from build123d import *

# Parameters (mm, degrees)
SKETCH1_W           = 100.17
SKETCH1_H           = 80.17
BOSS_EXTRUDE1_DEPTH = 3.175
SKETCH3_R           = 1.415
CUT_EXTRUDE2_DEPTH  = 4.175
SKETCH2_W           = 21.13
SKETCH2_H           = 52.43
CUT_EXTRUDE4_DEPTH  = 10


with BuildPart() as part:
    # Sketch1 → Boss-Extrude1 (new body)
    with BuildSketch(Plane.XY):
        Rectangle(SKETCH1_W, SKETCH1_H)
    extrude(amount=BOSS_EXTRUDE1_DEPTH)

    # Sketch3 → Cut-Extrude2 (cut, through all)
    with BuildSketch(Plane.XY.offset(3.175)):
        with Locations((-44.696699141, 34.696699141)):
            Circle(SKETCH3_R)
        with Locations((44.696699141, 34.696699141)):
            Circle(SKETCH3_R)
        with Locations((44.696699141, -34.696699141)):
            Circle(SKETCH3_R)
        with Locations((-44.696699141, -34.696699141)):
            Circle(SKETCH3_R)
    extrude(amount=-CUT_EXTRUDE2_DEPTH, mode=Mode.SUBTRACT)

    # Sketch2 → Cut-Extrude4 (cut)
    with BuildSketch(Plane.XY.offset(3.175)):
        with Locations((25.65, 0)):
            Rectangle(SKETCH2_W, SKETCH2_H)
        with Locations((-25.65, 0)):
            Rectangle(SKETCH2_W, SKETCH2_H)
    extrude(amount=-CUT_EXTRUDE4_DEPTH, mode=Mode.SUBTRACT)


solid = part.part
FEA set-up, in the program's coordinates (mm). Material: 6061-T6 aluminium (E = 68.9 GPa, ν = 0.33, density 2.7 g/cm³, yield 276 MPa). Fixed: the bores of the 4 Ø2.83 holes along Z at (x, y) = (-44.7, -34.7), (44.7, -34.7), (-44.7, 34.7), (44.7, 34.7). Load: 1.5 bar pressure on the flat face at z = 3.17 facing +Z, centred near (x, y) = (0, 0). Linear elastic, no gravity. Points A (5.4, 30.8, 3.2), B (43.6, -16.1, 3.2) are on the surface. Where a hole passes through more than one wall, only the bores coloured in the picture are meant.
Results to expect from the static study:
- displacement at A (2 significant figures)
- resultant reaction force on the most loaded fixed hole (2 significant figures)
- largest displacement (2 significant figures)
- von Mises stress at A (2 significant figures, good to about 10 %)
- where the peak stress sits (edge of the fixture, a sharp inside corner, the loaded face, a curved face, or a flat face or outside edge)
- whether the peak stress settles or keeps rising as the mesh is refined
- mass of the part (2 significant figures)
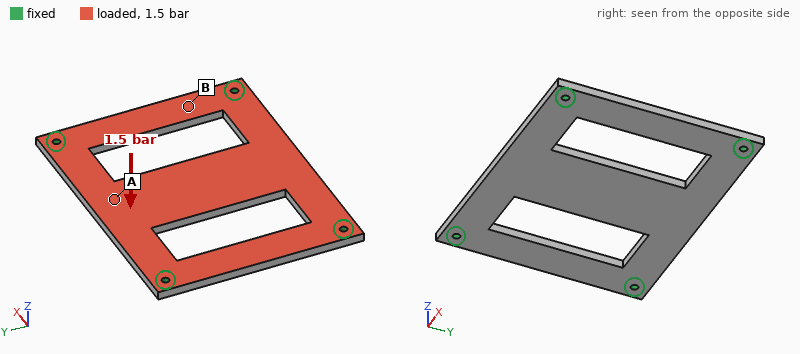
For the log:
0.23 mm
220 N
0.32 mm
37 MPa
edge of the fixture
keeps rising
50 g
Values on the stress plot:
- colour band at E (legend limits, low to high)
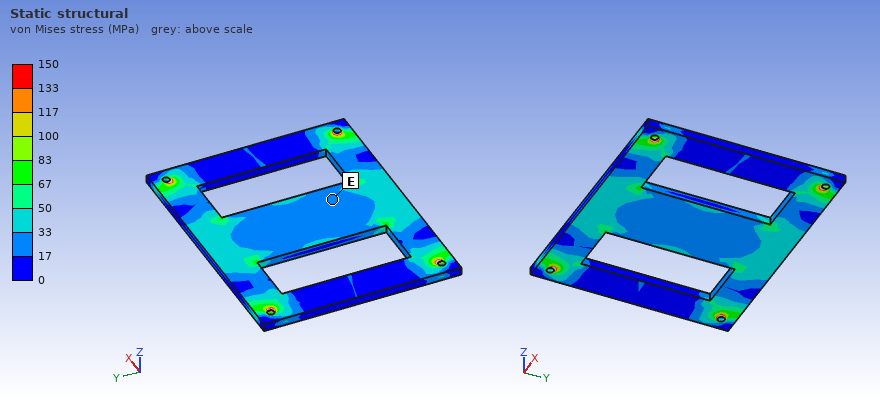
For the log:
17 to 33 MPa
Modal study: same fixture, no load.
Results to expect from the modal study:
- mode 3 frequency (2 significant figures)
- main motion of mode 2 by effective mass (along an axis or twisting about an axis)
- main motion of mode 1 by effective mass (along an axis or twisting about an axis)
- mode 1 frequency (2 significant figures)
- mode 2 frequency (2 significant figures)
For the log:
3300 Hz
twisting about X
along Z
1300 Hz
2100 Hz
